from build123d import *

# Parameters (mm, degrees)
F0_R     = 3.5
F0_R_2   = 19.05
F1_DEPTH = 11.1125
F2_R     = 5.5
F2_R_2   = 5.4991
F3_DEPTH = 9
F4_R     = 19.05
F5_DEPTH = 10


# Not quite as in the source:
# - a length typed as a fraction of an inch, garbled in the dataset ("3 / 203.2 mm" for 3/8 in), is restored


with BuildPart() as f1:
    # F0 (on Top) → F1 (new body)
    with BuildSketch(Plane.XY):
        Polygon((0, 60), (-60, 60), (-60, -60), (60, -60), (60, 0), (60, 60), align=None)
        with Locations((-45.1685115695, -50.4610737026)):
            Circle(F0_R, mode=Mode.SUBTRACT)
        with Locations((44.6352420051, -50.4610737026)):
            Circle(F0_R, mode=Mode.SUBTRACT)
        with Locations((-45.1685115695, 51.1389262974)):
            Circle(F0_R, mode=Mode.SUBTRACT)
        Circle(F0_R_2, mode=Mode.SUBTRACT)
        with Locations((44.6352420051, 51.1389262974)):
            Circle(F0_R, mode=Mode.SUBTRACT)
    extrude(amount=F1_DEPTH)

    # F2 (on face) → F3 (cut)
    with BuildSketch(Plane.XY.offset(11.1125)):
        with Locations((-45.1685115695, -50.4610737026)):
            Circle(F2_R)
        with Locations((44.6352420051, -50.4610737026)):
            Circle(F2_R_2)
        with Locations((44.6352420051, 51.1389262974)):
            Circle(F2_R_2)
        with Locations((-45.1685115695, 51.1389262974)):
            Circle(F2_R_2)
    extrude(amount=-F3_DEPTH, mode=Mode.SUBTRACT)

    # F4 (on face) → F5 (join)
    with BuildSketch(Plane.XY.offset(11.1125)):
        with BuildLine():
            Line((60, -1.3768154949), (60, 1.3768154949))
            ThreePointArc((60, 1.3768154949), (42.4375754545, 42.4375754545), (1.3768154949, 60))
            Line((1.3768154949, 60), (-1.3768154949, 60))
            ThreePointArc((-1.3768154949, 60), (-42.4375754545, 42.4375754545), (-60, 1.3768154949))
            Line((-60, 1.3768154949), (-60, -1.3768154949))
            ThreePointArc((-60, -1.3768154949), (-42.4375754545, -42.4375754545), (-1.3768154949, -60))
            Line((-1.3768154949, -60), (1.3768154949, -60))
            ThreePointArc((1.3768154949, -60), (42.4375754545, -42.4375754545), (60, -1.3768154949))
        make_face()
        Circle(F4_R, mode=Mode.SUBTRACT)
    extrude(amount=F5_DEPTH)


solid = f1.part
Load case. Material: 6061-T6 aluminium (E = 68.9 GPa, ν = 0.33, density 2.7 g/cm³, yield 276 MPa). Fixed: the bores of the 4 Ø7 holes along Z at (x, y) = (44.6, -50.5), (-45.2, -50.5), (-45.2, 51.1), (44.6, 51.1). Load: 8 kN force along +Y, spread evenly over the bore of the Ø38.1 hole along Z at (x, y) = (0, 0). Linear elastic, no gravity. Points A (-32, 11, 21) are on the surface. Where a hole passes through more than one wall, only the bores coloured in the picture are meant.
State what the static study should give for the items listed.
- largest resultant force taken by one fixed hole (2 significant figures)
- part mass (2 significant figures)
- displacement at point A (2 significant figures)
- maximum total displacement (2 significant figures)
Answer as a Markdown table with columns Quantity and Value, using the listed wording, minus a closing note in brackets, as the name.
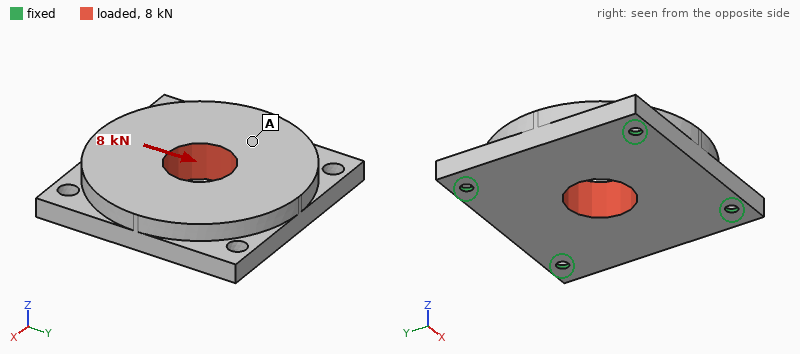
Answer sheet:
| Quantity | Value |
|---|---|
| largest resultant force taken by one fixed hole | 2.1 kN |
| part mass | 660 g |
| displacement at point A | 6.7 µm |
| maximum total displacement | 9.3 µm |
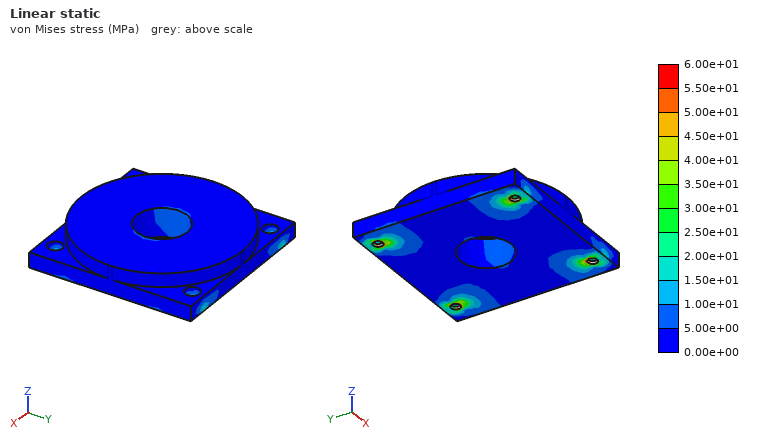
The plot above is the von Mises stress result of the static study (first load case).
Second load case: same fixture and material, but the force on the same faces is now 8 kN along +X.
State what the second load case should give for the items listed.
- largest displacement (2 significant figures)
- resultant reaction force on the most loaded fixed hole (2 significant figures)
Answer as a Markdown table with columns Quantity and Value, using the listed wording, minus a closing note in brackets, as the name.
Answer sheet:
| Quantity | Value |
|---|---|
| largest displacement | 10 µm |
| resultant reaction force on the most loaded fixed hole | 2.1 kN |
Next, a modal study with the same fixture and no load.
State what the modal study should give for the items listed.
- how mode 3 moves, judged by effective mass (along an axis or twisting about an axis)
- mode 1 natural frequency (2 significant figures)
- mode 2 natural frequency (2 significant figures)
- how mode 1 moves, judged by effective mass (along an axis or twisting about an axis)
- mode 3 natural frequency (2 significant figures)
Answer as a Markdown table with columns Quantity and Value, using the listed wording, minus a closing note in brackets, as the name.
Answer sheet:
| Quantity | Value |
|---|---|
| how mode 3 moves, judged by effective mass | twisting about X |
| mode 1 natural frequency | 3900 Hz |
| mode 2 natural frequency | 5200 Hz |
| how mode 1 moves, judged by effective mass | along Z |
| mode 3 natural frequency | 6200 Hz |
